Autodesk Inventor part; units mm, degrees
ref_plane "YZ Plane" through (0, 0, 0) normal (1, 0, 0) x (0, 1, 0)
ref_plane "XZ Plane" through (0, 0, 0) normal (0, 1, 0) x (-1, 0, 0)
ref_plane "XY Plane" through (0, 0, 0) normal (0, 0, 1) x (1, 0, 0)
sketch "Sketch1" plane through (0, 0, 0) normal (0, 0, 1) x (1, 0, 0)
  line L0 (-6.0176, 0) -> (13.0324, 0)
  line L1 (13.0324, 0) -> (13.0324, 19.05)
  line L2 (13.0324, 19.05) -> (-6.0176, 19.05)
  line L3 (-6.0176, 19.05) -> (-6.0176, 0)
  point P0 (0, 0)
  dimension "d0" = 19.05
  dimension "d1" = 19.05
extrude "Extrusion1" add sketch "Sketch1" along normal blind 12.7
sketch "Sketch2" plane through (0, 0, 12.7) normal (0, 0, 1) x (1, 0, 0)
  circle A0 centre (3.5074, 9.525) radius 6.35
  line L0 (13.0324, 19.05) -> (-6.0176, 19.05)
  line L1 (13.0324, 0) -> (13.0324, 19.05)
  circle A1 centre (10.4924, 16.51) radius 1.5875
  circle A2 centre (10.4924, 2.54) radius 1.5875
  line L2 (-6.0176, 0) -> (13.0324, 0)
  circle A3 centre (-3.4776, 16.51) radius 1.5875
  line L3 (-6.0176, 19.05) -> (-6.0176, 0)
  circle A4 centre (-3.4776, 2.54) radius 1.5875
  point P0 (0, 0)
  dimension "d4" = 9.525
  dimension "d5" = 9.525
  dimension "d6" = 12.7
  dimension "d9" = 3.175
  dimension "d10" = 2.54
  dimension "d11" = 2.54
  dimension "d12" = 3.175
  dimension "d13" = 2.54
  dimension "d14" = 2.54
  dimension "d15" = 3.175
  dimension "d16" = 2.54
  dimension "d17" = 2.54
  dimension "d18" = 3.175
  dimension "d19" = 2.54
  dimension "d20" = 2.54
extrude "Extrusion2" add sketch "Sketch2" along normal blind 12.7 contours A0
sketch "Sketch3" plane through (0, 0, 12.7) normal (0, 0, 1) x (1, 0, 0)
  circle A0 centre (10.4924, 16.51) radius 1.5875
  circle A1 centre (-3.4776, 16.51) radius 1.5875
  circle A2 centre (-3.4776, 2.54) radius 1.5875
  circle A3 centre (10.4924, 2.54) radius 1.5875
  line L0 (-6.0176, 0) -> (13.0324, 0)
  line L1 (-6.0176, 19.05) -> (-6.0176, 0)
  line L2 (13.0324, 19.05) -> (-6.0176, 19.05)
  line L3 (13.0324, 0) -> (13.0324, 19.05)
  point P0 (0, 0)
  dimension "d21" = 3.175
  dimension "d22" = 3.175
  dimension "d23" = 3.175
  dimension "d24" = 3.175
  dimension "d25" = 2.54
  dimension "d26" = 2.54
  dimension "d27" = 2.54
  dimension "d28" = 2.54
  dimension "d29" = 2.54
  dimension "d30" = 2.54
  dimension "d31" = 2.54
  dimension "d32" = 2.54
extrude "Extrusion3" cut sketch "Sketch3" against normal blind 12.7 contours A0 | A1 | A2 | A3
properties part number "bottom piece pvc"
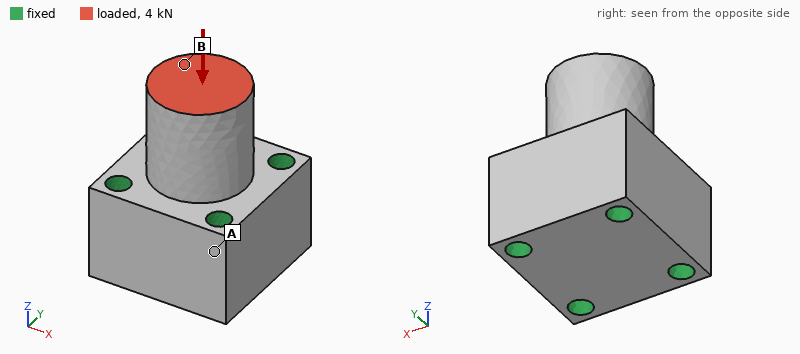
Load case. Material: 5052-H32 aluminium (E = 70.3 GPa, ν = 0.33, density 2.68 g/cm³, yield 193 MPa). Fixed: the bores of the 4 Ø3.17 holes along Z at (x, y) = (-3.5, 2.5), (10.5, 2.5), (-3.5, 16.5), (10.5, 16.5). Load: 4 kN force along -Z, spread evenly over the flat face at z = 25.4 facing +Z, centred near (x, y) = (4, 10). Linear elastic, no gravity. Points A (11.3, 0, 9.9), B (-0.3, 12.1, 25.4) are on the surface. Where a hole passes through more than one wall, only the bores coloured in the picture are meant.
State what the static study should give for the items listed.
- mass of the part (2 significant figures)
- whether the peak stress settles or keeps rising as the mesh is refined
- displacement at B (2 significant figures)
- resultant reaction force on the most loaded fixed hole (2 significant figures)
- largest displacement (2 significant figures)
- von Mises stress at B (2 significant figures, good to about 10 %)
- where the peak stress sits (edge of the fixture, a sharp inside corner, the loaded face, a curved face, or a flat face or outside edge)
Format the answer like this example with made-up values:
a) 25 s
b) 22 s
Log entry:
a) 16 g
b) keeps rising
c) 8.3 µm
d) 1.1 kN
e) 8.4 µm
f) 32 MPa
g) edge of the fixture
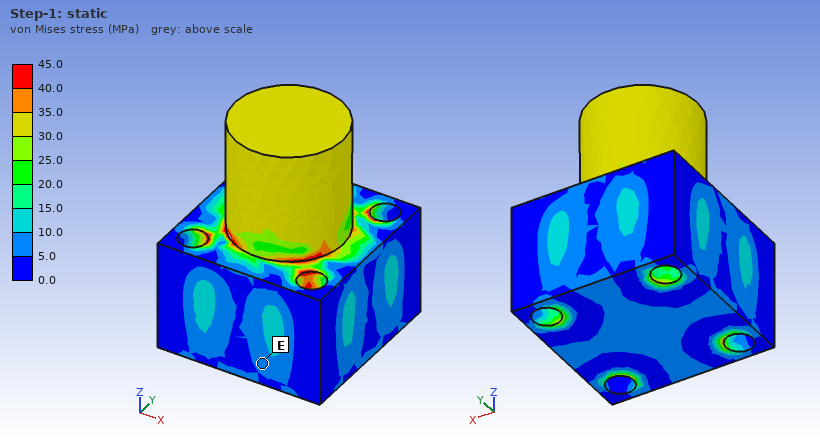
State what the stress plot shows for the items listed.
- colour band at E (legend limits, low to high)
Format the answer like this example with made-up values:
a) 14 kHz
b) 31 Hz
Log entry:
a) 5.0 to 10.0 MPa
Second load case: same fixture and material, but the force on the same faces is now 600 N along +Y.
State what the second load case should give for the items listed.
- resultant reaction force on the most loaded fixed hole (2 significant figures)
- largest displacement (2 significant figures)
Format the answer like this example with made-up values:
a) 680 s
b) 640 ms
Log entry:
a) 390 N
b) 12 µm
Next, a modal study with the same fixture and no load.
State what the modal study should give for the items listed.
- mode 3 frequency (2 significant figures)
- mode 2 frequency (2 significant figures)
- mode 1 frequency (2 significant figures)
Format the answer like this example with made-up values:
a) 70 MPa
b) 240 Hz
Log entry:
a) 54 kHz
b) 30 kHz
c) 30 kHz
